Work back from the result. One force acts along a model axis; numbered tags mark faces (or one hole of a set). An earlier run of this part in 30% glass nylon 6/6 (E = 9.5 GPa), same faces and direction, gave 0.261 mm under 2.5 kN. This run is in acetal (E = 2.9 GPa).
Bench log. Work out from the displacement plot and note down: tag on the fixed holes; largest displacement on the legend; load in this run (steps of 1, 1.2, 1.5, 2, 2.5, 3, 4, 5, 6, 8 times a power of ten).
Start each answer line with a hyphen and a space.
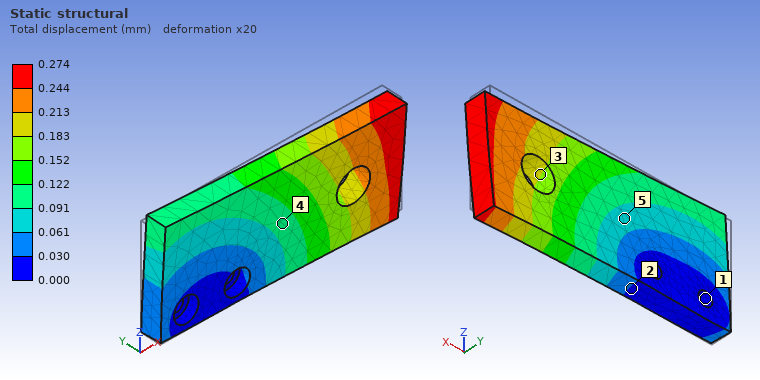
- 1
- 0.274 mm
- 800 N
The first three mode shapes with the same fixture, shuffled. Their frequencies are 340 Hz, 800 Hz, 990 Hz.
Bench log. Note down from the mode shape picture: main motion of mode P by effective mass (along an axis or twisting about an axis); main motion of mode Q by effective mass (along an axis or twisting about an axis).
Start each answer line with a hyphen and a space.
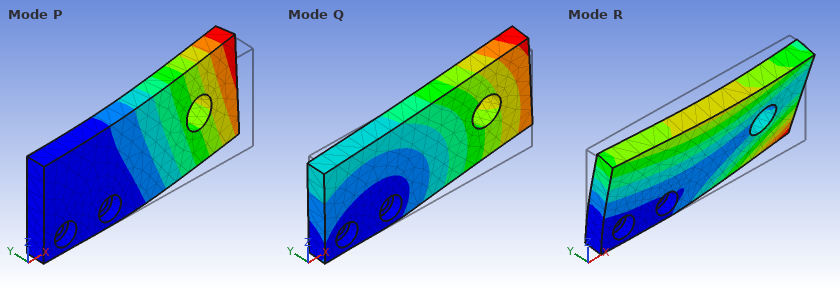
- along Y
- along Z
